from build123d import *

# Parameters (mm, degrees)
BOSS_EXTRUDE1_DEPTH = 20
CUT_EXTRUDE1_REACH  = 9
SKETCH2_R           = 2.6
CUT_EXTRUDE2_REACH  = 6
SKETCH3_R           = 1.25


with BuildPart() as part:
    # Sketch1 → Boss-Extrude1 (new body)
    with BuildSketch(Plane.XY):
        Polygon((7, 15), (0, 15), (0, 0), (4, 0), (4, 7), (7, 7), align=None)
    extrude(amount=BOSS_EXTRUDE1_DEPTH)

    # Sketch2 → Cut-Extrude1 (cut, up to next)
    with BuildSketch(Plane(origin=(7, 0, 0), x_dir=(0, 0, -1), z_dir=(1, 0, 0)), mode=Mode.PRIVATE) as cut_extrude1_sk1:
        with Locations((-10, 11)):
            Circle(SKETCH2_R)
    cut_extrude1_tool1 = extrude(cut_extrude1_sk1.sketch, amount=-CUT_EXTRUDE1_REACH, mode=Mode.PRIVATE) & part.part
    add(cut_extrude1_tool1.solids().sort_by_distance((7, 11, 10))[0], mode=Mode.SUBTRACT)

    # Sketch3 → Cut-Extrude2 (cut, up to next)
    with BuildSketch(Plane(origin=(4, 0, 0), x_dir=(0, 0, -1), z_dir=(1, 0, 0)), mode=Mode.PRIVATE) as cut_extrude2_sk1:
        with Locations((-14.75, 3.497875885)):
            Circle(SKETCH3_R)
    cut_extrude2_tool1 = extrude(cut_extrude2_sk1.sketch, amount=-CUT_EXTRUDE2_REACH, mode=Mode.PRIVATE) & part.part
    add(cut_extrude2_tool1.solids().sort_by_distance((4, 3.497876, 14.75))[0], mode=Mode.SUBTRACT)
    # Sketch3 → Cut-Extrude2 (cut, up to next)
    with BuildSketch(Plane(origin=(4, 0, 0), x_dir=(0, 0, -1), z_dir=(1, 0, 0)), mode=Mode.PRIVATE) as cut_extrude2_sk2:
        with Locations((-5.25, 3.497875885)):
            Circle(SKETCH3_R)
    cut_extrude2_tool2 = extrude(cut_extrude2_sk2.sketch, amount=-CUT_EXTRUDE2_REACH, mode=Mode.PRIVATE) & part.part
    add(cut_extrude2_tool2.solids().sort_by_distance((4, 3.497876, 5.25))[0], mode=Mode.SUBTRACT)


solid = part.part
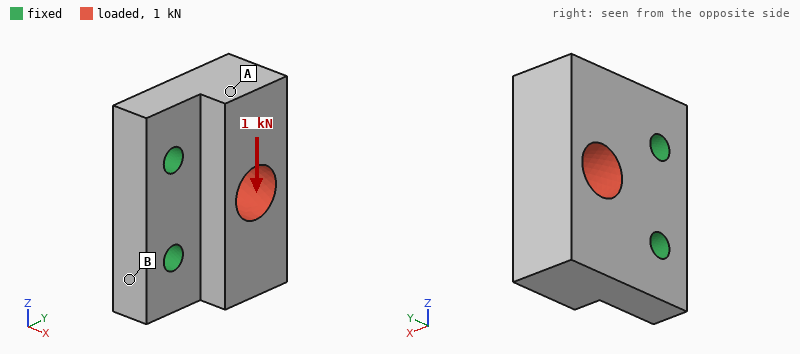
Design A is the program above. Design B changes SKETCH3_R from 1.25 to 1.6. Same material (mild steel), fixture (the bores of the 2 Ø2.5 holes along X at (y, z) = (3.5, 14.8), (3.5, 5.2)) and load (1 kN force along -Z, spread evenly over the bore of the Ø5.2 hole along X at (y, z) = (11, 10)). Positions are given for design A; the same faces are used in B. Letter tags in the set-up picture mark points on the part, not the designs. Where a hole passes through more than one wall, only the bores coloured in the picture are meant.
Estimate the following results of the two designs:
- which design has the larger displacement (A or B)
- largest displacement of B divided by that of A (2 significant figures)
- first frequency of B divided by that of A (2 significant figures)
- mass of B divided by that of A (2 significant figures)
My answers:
A
0.87
1.1
0.98
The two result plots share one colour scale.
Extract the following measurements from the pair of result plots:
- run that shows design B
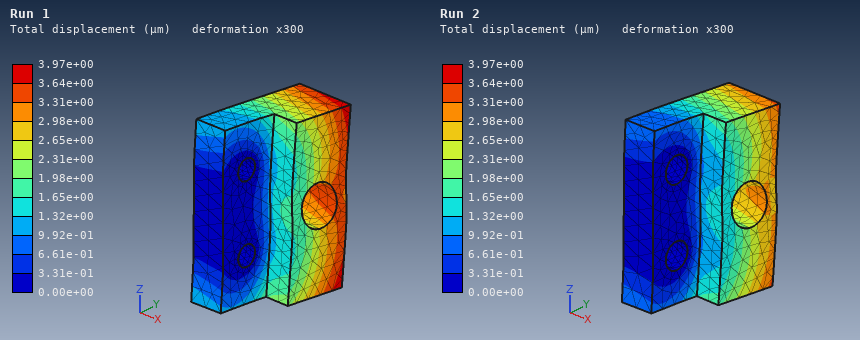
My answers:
Run 2
